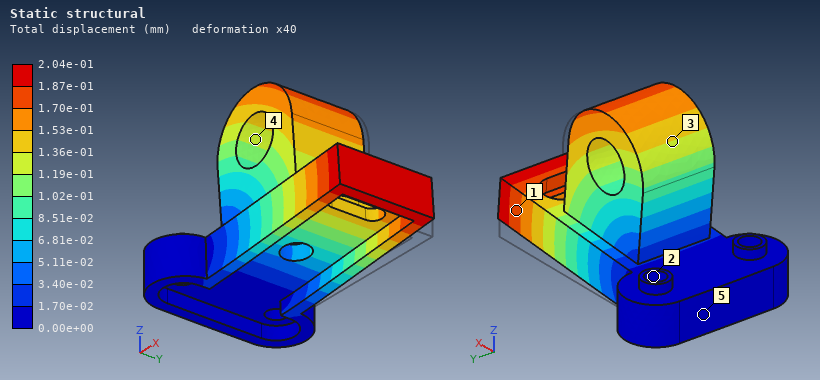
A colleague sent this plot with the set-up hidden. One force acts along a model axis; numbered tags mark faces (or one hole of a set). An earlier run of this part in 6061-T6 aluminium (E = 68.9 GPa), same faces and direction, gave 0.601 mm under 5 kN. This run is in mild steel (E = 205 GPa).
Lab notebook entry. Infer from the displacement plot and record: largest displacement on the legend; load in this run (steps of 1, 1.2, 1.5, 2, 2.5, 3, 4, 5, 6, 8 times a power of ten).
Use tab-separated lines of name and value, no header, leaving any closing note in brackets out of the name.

largest displacement on the legend	2.04e-01 mm
load in this run	5 kN
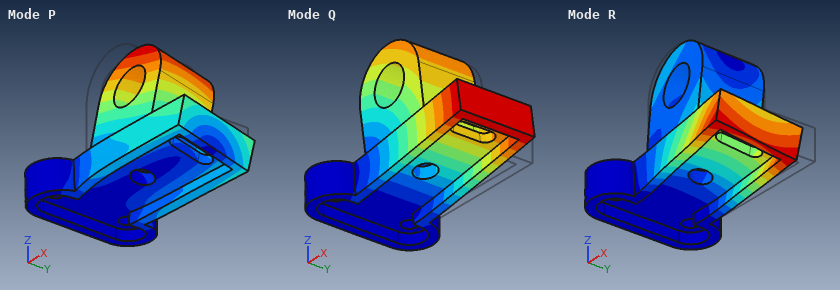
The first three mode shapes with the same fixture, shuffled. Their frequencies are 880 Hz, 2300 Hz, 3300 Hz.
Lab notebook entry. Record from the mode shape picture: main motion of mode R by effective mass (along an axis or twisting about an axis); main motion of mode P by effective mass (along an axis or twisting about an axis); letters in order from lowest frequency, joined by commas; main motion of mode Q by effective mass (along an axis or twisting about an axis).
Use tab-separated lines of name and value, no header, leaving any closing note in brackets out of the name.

main motion of mode R by effective mass	along Y
main motion of mode P by effective mass	along Y
letters in order from lowest frequency, joined by commas	Q, P, R
main motion of mode Q by effective mass	along Z
